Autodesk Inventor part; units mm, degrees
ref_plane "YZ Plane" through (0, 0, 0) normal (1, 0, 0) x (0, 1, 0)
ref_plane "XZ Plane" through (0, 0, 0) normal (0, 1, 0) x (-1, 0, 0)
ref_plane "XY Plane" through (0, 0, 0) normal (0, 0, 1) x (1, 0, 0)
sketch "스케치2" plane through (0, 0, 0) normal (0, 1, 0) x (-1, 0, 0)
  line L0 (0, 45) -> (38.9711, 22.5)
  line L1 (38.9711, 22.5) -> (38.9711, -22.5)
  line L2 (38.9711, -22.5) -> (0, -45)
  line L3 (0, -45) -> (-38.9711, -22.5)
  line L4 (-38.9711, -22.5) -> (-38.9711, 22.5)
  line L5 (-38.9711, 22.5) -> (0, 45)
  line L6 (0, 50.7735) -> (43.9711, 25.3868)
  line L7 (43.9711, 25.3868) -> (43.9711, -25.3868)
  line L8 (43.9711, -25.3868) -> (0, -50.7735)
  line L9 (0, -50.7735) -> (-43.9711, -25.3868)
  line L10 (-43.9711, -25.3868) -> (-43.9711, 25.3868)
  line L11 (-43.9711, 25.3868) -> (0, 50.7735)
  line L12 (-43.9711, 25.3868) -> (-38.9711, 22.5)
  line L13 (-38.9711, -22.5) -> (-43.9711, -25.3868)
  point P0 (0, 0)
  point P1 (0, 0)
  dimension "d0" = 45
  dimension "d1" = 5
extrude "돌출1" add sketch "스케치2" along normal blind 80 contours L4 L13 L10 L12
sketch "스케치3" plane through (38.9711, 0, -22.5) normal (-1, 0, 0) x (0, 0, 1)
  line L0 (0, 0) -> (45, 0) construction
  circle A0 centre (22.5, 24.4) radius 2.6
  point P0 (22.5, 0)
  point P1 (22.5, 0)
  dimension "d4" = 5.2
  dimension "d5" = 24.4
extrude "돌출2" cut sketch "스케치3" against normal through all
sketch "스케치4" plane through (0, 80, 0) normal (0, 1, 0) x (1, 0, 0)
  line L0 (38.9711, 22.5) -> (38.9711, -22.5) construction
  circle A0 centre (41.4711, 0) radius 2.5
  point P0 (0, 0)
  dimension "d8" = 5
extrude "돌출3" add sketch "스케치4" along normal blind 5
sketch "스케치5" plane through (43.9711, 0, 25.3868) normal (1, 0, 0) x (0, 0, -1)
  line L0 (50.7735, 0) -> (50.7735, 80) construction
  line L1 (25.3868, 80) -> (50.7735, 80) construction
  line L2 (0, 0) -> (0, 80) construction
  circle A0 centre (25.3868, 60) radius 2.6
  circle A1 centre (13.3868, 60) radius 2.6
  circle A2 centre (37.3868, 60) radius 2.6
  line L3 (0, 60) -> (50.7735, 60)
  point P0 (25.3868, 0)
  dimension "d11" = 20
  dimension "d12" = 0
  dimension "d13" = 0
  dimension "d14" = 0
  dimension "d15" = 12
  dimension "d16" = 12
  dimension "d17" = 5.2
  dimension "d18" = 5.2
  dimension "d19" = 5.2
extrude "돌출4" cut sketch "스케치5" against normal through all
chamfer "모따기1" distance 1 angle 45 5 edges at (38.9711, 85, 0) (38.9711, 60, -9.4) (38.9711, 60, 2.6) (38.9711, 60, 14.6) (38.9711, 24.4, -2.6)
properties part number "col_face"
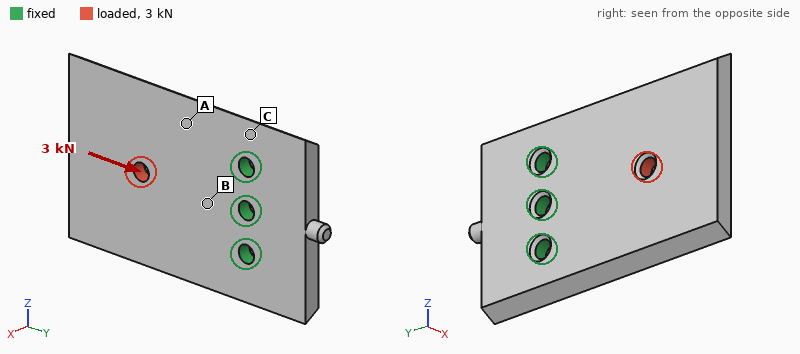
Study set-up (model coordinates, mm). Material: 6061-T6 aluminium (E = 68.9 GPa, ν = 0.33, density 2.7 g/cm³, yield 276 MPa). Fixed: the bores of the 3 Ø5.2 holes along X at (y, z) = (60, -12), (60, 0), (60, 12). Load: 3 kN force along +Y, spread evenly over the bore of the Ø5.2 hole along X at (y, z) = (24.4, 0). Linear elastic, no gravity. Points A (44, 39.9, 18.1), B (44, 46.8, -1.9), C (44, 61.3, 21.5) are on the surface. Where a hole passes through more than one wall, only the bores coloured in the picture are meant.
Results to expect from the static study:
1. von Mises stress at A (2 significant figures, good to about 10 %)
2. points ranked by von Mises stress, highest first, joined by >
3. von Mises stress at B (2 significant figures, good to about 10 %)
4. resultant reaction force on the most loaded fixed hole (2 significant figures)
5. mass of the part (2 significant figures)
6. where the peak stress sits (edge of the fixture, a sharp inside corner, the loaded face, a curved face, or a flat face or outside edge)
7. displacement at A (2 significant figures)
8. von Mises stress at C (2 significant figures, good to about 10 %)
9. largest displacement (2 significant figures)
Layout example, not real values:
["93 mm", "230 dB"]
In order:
["15 MPa", "B > A > C", "24 MPa", "1.1 kN", "51 g", "the loaded face", "8.6 µm", "6.9 MPa", "56 µm"]
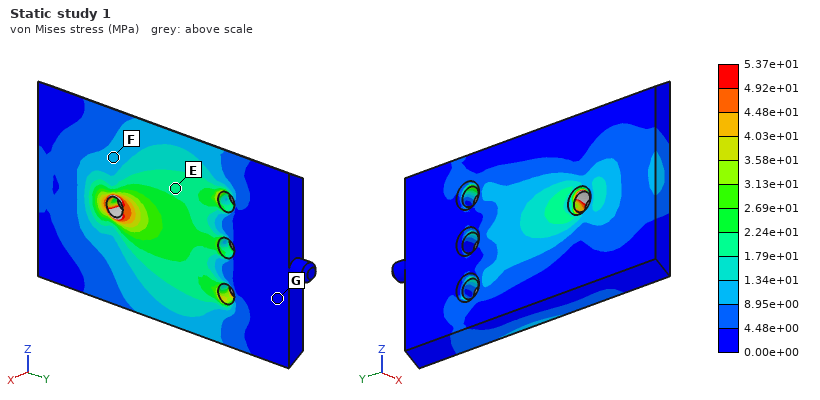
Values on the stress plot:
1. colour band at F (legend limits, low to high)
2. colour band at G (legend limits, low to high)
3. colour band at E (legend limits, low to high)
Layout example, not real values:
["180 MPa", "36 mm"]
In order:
["8.95e+00 to 1.34e+01 MPa", "0.00e+00 to 4.48e+00 MPa", "1.79e+01 to 2.24e+01 MPa"]
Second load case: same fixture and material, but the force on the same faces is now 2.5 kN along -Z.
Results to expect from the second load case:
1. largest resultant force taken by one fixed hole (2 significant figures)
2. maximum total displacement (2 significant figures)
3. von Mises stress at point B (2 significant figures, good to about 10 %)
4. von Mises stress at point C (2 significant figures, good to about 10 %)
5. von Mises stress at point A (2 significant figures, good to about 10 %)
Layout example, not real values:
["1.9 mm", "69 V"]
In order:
["3.3 kN", "66 µm", "37 MPa", "17 MPa", "22 MPa"]
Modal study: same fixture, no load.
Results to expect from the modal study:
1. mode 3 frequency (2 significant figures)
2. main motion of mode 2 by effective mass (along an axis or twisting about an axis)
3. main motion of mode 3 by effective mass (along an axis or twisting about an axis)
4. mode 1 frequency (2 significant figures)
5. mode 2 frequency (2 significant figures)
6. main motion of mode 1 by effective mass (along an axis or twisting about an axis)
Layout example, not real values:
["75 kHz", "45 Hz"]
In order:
["6700 Hz", "twisting about Y", "along Z", "1200 Hz", "3100 Hz", "along X"]
